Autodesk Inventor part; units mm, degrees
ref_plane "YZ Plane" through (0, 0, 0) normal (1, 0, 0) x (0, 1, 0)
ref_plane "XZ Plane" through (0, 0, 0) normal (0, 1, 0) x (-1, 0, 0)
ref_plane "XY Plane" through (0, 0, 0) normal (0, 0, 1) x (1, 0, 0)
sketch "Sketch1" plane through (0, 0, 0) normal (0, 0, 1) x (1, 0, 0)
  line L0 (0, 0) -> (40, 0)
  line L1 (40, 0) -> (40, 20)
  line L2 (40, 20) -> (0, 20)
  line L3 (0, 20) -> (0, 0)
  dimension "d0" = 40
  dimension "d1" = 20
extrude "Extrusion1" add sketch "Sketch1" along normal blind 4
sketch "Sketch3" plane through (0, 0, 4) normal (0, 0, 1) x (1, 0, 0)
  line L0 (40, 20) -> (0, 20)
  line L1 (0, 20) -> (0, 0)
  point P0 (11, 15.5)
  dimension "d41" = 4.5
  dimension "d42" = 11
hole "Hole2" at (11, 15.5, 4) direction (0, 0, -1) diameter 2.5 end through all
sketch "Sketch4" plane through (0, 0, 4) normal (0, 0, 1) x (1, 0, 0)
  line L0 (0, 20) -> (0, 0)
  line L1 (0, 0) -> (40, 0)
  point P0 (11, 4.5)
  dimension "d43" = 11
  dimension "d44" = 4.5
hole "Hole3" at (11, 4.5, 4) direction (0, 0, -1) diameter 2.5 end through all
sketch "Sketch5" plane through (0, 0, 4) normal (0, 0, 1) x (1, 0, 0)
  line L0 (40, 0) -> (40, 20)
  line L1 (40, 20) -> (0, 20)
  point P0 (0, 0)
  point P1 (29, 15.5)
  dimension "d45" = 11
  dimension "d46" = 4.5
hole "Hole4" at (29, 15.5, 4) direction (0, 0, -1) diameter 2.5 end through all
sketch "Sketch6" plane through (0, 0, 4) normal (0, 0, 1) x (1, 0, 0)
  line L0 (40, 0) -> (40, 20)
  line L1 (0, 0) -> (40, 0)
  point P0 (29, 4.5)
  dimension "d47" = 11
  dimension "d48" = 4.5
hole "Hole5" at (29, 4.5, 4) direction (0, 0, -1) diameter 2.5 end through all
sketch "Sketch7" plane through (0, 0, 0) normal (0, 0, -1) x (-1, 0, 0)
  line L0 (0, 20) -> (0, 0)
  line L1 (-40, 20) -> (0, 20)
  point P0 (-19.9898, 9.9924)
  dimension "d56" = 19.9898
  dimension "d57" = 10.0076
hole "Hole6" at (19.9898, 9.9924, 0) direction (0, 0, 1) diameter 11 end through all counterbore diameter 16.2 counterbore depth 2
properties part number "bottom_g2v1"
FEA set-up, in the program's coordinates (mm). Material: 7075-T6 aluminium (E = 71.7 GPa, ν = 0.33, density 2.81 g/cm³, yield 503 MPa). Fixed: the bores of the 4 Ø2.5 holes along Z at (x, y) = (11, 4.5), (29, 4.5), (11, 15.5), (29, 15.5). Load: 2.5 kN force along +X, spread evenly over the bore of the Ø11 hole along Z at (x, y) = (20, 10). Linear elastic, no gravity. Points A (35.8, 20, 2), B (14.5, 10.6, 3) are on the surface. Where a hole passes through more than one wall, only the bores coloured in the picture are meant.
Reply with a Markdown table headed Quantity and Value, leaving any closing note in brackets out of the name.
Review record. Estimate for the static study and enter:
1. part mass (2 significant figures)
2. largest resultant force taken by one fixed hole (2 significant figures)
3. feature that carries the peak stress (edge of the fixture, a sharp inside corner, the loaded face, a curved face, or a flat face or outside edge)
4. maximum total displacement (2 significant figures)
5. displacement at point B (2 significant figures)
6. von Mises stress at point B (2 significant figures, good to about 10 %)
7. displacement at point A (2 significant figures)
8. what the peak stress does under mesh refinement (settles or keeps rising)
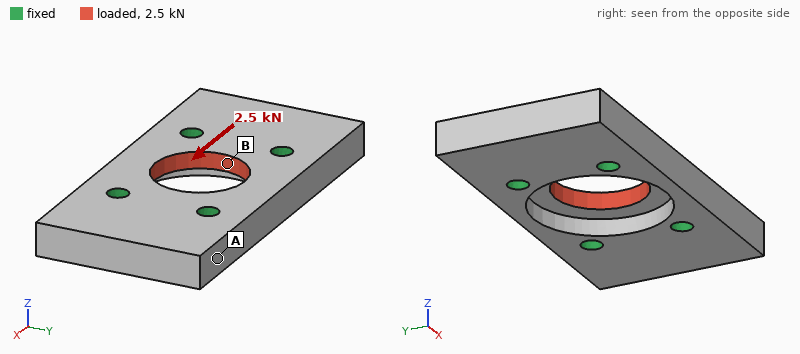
| Quantity | Value |
|---|---|
| part mass | 7.1 g |
| largest resultant force taken by one fixed hole | 640 N |
| feature that carries the peak stress | edge of the fixture |
| maximum total displacement | 4.0 µm |
| displacement at point B | 3.2 µm |
| von Mises stress at point B | 33 MPa |
| displacement at point A | 0.63 µm |
| what the peak stress does under mesh refinement | keeps rising |
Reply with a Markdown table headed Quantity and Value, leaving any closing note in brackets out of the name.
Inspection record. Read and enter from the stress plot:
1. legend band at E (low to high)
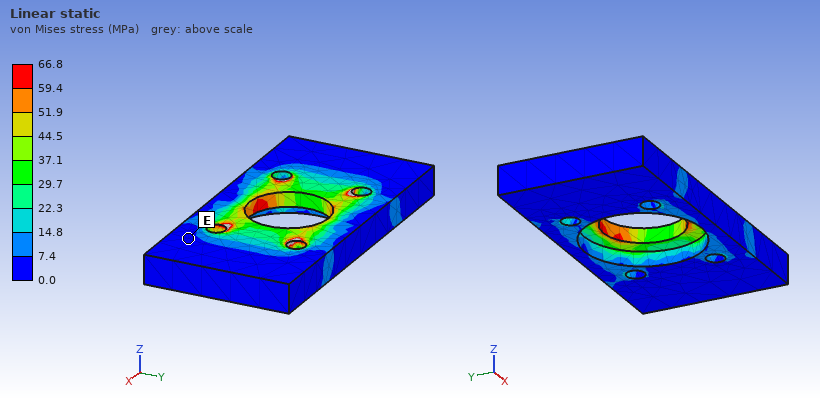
| Quantity | Value |
|---|---|
| legend band at E | 0.0 to 7.4 MPa |
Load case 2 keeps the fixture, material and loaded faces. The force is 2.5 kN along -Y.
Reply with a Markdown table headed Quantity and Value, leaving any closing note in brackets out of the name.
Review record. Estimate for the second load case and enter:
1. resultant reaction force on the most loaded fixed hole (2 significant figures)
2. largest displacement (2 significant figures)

| Quantity | Value |
|---|---|
| resultant reaction force on the most loaded fixed hole | 640 N |
| largest displacement | 11 µm |
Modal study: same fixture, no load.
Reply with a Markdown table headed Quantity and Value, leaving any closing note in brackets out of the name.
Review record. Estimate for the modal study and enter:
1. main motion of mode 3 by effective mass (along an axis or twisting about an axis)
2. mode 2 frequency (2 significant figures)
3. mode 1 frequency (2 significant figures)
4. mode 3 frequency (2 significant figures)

| Quantity | Value |
|---|---|
| main motion of mode 3 by effective mass | twisting about X |
| mode 2 frequency | 24 kHz |
| mode 1 frequency | 24 kHz |
| mode 3 frequency | 36 kHz |
